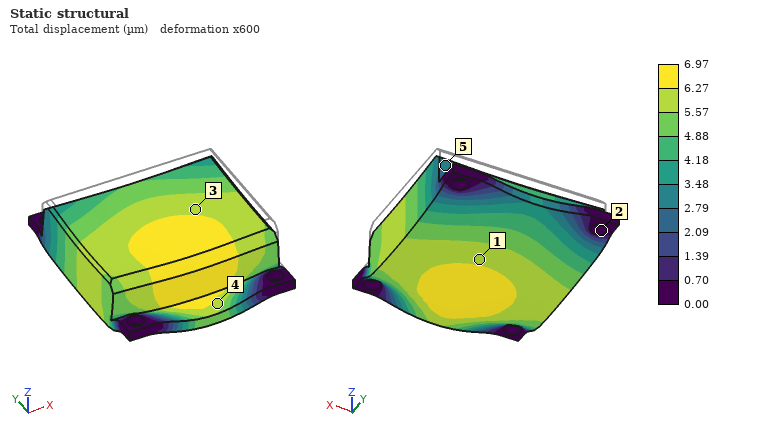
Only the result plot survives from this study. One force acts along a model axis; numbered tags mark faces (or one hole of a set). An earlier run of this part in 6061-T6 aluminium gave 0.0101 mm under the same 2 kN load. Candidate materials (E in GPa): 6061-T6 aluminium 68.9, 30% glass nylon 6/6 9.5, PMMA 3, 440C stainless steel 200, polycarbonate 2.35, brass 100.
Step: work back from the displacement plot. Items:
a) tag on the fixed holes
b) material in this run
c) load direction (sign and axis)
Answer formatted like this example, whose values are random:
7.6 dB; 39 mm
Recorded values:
2; brass; -Z
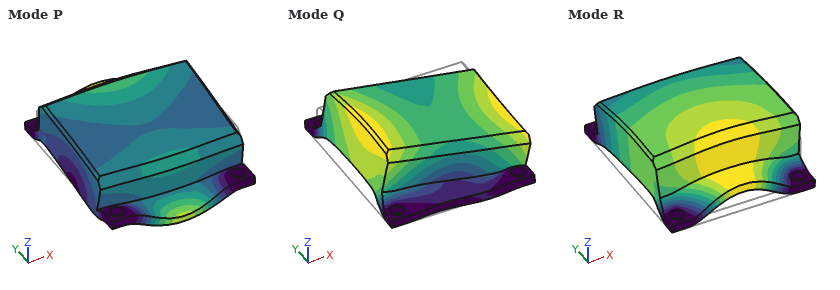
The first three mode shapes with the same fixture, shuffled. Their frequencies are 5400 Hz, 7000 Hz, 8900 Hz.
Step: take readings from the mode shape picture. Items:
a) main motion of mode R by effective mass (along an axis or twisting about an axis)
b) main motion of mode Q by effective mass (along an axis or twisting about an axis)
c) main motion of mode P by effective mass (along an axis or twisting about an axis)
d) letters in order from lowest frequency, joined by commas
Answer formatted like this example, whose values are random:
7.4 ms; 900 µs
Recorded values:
along Z; along X; along Y; R, Q, P
